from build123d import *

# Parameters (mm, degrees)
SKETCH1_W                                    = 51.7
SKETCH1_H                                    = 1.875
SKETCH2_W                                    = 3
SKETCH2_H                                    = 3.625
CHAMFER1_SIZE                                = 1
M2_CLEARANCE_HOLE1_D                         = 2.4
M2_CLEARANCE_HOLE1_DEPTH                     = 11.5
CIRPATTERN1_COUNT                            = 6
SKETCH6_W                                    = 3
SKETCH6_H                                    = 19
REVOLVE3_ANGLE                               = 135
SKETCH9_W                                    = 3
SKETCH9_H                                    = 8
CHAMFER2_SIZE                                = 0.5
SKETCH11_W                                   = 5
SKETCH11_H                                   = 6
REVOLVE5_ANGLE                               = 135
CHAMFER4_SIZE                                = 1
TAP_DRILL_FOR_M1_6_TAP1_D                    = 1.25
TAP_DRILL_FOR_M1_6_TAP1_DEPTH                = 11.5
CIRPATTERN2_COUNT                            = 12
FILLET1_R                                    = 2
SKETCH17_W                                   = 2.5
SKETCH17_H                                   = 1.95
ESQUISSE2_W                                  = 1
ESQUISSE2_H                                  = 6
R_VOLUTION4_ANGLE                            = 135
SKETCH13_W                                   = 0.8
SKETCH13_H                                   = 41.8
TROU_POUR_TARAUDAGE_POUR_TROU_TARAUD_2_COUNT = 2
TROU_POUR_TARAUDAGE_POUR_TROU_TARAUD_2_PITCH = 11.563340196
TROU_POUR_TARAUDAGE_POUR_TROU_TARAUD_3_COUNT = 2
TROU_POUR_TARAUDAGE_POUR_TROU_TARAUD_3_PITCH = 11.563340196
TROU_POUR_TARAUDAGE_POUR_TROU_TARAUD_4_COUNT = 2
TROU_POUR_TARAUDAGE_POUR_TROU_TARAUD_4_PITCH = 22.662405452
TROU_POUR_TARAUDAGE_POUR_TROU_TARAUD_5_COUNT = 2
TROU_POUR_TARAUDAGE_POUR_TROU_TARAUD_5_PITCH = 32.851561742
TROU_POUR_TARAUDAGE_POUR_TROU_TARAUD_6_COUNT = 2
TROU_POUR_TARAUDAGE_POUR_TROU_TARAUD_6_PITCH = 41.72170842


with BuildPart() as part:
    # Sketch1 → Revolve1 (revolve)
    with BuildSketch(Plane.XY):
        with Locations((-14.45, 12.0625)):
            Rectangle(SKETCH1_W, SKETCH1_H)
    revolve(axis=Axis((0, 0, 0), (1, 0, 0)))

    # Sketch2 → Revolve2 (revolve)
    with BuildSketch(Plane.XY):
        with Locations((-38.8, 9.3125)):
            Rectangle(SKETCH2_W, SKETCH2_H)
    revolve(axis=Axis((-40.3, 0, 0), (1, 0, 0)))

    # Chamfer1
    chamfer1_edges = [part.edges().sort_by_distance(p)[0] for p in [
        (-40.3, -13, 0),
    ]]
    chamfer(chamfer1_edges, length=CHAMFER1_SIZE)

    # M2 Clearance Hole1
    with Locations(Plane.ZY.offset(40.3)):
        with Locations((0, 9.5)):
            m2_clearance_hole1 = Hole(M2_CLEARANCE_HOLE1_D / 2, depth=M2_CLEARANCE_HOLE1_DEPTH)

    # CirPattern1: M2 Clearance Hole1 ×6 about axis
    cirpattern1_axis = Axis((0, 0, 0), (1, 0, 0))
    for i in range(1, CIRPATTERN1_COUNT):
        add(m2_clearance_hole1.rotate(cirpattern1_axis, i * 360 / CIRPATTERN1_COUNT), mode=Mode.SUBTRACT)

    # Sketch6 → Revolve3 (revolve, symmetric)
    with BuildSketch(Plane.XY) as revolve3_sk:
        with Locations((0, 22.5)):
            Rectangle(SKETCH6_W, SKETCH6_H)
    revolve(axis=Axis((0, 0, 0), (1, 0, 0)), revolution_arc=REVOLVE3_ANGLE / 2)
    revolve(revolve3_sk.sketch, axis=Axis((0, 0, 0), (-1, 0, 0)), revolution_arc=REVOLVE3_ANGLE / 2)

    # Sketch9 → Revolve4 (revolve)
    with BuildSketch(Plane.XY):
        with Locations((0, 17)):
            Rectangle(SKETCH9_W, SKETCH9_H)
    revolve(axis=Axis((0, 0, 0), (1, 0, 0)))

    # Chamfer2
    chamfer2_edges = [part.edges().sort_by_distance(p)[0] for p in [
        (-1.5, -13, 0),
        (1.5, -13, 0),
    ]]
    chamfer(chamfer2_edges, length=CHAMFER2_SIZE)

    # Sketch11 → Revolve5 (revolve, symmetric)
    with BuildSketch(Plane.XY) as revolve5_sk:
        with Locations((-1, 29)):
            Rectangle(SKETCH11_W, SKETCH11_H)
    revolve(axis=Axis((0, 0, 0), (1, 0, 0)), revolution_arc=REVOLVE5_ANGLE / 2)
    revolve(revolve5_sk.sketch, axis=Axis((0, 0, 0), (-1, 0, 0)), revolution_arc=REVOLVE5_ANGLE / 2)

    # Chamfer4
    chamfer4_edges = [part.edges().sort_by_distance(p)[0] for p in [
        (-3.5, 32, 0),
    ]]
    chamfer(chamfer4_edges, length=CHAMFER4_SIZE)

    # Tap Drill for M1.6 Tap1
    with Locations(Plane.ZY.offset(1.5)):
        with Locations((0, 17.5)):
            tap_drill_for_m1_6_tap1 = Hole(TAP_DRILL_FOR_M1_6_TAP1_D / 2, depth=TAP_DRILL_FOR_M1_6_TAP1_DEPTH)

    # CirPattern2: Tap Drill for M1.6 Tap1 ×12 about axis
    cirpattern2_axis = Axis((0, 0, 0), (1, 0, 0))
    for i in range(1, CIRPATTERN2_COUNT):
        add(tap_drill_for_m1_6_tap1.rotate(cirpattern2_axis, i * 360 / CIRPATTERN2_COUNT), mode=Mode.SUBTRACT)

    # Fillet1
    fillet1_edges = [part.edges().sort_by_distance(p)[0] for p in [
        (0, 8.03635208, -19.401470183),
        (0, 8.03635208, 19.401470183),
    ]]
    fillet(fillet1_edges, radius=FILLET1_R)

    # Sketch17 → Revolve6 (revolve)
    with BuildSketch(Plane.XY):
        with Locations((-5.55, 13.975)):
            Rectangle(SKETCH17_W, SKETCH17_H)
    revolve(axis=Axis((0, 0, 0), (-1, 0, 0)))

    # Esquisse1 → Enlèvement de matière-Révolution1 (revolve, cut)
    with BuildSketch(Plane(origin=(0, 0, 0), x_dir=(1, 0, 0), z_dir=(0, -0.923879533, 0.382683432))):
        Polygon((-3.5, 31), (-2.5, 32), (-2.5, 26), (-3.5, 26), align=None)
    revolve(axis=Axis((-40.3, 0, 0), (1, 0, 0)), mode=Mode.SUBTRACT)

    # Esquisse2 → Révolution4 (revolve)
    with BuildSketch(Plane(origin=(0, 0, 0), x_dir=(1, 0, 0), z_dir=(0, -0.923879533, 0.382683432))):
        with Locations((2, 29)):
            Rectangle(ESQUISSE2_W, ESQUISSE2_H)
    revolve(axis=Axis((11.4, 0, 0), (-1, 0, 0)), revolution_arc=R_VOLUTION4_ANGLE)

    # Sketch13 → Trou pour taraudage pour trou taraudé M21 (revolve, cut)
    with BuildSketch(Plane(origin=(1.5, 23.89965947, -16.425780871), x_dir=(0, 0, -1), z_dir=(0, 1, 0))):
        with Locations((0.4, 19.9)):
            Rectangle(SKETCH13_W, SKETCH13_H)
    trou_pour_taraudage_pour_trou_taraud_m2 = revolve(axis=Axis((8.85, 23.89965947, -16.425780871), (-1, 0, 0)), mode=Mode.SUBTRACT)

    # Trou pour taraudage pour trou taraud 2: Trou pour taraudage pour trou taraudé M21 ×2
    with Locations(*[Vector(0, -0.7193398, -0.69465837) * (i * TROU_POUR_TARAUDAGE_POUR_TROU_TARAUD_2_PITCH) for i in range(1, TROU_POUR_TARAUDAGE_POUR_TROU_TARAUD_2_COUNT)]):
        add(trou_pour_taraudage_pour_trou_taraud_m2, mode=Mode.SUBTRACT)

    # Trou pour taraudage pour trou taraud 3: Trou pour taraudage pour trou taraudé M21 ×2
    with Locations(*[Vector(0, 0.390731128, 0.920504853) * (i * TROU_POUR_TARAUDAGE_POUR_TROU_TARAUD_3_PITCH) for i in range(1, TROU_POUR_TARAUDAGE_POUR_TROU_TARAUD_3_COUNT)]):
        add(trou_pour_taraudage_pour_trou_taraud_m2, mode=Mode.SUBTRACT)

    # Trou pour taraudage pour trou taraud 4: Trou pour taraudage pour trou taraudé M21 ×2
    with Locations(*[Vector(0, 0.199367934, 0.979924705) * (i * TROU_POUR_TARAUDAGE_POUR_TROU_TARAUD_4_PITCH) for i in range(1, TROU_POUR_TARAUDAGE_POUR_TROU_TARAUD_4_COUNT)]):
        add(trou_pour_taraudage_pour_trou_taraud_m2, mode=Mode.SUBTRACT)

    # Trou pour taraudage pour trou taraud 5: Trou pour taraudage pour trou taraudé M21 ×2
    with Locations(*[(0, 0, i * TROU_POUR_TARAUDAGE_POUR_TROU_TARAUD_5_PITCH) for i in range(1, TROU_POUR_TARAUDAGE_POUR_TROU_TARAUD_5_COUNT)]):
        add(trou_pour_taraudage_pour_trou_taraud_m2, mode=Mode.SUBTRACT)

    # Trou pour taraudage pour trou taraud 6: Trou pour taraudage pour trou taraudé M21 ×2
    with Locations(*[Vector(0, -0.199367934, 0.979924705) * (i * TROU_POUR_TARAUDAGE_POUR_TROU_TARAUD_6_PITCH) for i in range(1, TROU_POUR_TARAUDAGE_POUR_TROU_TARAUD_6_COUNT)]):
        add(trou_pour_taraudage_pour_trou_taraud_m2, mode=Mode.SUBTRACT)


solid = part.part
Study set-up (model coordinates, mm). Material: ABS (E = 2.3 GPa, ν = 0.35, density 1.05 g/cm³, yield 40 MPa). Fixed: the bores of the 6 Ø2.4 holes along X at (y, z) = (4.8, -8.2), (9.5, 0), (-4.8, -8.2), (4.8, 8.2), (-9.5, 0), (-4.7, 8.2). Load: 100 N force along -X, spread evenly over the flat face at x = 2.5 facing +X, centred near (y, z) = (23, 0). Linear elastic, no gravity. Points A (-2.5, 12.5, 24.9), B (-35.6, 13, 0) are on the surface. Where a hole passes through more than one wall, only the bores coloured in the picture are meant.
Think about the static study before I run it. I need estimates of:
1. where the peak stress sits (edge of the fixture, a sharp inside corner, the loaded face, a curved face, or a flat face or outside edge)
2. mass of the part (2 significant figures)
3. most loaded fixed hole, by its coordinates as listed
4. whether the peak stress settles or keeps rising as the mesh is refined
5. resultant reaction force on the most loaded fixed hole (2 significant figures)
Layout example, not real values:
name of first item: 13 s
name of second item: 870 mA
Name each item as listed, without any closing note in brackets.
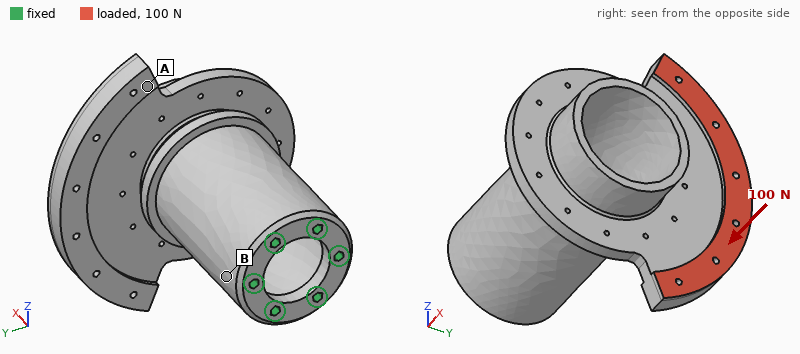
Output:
where the peak stress sits: edge of the fixture
mass of the part: 14 g
most loaded fixed hole, by its coordinates as listed: (9.5, 0)
whether the peak stress settles or keeps rising as the mesh is refined: keeps rising
resultant reaction force on the most loaded fixed hole: 76 N
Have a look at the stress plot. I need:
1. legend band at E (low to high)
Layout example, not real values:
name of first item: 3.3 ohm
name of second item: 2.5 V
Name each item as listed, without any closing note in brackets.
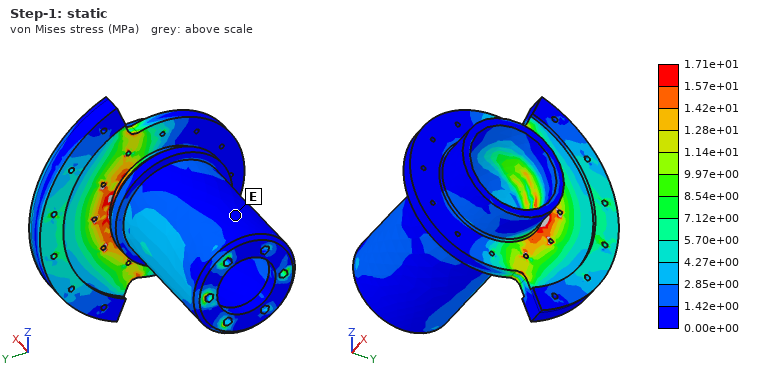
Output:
legend band at E: 0.00e+00 to 1.42e+00 MPa
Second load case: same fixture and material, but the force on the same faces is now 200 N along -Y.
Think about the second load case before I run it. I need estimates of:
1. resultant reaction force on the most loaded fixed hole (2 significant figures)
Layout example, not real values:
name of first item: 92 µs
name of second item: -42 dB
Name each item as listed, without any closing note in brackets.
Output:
resultant reaction force on the most loaded fixed hole: 220 N
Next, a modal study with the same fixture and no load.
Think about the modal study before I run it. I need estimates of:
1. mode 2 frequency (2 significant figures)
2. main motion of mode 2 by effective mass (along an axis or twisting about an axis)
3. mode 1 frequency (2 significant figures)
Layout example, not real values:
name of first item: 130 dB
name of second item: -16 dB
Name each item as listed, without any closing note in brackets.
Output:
mode 2 frequency: 990 Hz
main motion of mode 2 by effective mass: along Z
mode 1 frequency: 950 Hz
